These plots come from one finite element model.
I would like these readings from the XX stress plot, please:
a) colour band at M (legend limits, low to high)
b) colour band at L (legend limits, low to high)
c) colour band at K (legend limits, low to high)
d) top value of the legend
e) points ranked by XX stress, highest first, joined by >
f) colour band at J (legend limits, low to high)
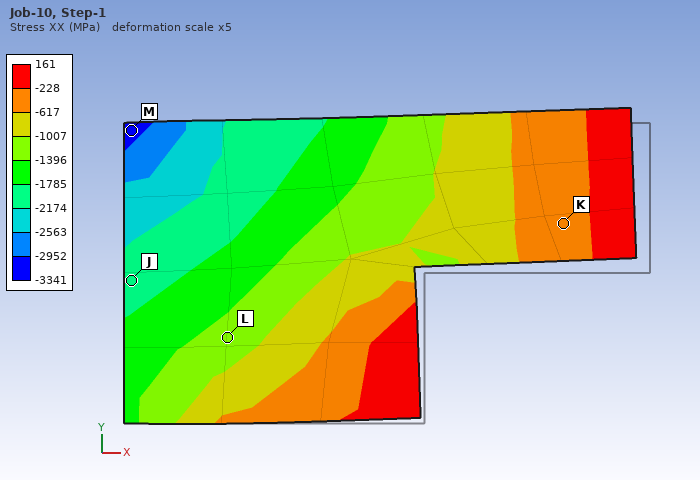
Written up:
-3341 to -2952 MPa
-1396 to -1007 MPa
-617 to -228 MPa
161 MPa
K > L > J > M
-2174 to -1785 MPa
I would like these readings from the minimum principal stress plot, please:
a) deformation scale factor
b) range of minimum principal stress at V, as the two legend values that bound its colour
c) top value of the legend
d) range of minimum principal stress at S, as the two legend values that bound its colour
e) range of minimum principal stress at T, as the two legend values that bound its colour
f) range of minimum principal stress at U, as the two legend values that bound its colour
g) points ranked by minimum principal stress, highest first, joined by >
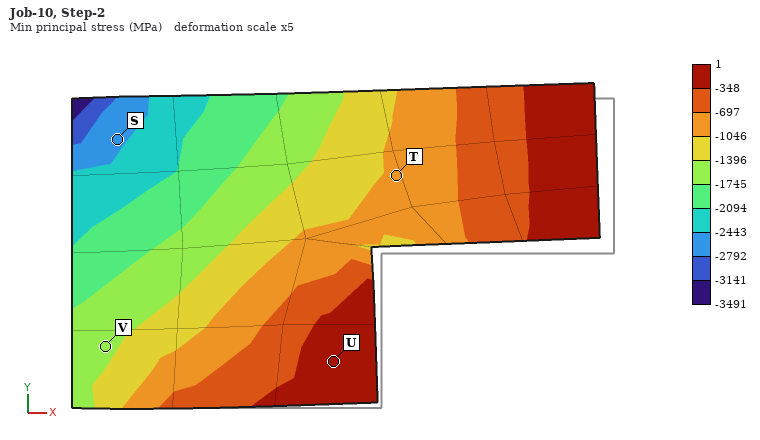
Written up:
5
-1745 to -1396 MPa
1 MPa
-2792 to -2443 MPa
-1046 to -697 MPa
-348 to 1 MPa
U > T > V > S
